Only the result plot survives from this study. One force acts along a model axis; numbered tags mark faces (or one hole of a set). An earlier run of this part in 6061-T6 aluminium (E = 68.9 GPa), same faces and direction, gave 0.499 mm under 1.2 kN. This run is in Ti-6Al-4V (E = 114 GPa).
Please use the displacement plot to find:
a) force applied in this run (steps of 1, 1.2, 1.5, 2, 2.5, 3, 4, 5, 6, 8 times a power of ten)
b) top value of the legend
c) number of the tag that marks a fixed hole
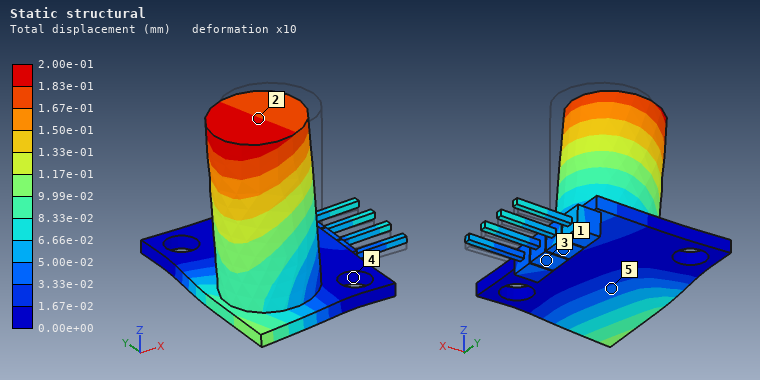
800 N
2.00e-01 mm
4
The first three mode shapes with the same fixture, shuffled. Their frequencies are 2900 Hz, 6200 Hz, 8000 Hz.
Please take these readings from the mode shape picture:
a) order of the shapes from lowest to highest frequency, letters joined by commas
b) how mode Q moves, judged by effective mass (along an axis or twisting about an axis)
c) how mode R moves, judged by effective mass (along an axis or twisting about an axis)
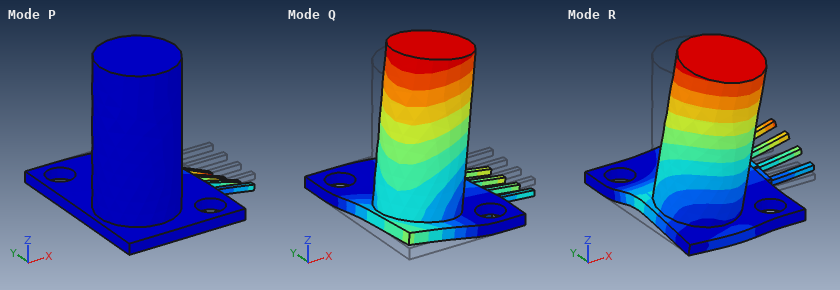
Q, R, P
along X
along Y
